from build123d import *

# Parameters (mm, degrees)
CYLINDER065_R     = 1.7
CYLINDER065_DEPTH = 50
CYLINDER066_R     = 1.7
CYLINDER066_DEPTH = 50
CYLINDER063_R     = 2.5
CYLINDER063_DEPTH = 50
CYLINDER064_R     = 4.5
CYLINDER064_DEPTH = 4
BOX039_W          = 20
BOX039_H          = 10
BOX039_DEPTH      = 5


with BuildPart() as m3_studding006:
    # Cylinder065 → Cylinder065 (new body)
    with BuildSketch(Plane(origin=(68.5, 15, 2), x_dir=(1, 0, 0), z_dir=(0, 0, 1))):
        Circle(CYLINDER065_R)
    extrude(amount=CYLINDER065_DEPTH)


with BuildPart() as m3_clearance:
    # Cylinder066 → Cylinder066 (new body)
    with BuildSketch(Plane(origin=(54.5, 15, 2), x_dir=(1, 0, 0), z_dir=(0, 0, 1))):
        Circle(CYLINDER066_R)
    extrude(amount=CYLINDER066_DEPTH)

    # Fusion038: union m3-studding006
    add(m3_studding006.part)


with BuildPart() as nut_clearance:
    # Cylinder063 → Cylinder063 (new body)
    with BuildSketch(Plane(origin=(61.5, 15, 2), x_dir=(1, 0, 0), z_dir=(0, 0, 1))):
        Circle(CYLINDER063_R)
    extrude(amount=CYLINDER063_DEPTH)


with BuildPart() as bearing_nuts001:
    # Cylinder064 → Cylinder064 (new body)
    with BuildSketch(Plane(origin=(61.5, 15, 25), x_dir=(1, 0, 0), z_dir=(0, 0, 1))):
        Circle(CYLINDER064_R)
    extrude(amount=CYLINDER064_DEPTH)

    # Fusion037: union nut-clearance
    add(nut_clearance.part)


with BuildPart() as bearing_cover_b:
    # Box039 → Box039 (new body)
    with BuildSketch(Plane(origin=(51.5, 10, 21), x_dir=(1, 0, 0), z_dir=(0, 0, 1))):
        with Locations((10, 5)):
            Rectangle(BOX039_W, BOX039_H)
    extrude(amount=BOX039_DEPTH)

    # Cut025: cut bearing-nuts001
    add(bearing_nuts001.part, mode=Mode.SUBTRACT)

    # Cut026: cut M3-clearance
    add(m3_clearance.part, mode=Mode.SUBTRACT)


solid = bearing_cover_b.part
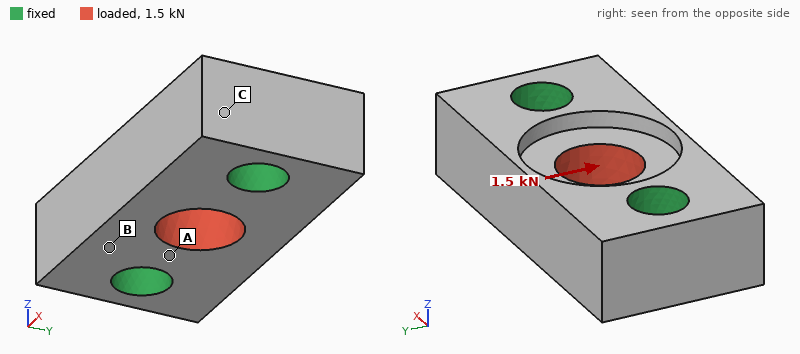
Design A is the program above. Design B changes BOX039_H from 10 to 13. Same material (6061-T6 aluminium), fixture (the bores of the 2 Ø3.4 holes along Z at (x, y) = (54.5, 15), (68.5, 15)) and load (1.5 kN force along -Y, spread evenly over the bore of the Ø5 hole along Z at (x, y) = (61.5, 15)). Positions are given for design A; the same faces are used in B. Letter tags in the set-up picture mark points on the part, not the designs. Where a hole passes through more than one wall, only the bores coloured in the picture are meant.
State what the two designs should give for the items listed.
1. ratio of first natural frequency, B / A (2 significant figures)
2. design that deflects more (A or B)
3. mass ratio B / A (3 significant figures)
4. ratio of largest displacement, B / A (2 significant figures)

0.73
A
1.39
0.73
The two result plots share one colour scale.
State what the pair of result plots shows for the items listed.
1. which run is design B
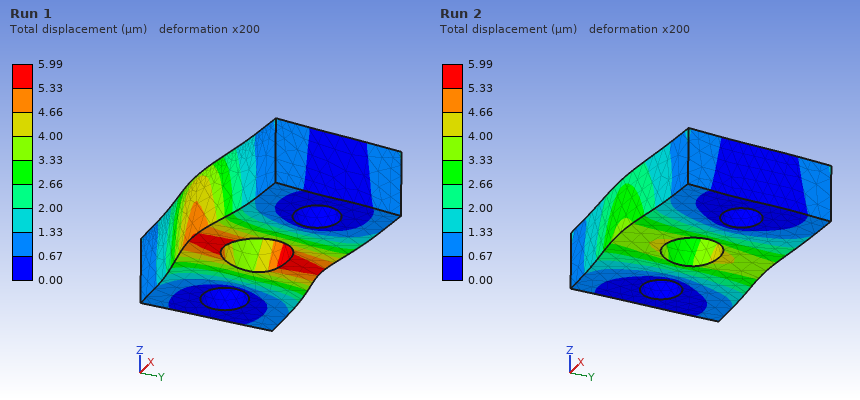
Run 2
